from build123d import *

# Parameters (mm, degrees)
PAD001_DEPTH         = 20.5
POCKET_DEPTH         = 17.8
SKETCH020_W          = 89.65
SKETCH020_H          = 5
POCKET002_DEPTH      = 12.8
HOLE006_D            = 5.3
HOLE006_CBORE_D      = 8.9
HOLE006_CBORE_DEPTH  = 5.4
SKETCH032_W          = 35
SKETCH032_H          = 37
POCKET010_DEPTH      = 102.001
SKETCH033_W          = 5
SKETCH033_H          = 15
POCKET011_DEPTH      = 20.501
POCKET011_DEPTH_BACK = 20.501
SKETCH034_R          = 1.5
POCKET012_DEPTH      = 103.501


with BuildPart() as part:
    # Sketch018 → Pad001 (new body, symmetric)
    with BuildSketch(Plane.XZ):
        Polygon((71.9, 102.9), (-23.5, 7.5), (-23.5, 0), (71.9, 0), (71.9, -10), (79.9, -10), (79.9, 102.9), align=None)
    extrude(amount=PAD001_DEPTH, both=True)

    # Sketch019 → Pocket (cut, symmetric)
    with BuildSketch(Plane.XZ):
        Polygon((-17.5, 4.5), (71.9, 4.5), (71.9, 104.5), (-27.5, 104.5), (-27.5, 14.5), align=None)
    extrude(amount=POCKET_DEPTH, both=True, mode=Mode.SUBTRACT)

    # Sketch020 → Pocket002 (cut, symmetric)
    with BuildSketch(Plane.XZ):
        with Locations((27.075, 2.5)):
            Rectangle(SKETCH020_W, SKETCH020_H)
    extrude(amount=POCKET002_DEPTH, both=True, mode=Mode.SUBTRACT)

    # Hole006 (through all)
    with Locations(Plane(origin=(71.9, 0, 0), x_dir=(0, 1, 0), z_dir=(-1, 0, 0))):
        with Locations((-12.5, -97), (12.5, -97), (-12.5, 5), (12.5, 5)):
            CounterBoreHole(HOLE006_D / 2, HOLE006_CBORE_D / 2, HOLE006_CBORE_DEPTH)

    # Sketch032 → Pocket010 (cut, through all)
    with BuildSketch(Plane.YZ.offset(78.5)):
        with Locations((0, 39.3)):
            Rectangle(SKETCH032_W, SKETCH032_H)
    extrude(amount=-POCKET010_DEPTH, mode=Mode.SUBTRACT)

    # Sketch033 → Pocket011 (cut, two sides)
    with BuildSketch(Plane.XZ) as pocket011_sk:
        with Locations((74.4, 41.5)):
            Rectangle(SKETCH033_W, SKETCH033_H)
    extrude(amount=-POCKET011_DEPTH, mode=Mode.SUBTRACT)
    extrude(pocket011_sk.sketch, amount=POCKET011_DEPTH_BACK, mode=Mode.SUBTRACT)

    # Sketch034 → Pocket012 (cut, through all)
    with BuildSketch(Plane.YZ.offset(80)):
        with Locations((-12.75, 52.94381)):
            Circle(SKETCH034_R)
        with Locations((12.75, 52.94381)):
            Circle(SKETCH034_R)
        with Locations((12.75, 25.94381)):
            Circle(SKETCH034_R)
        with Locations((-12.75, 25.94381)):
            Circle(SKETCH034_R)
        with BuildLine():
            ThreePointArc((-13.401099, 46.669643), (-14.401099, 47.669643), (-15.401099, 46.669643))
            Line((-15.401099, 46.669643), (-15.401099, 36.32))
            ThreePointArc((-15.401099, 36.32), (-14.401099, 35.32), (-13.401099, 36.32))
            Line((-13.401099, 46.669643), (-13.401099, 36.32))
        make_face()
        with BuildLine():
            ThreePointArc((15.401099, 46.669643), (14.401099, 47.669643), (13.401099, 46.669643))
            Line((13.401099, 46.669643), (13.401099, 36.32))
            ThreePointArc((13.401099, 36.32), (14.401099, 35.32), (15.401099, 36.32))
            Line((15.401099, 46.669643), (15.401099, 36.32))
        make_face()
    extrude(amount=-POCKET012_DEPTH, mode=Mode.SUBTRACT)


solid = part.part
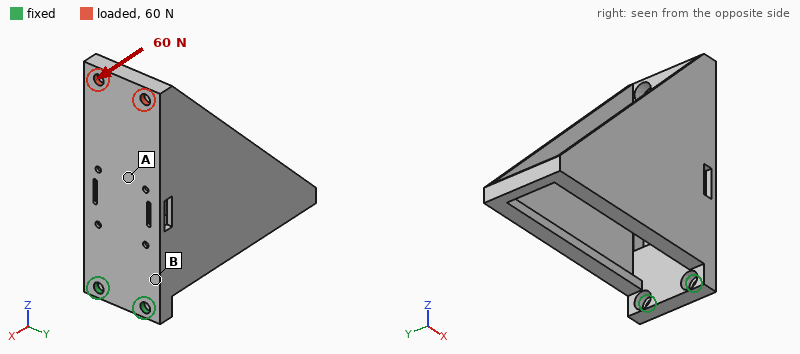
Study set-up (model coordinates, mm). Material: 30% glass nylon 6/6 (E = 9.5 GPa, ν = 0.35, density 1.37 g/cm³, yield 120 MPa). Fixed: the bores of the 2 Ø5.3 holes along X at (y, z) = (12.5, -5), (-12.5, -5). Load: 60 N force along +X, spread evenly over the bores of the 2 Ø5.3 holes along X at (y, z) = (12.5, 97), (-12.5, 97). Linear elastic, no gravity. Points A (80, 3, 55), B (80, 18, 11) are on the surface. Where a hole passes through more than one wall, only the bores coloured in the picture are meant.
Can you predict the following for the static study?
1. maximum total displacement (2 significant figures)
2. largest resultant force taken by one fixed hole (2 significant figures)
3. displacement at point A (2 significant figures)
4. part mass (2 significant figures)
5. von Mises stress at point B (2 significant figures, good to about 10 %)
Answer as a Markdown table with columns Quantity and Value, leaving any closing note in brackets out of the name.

| Quantity | Value |
|---|---|
| maximum total displacement | 1.5 mm |
| largest resultant force taken by one fixed hole | 51 N |
| displacement at point A | 0.82 mm |
| part mass | 83 g |
| von Mises stress at point B | 5.4 MPa |
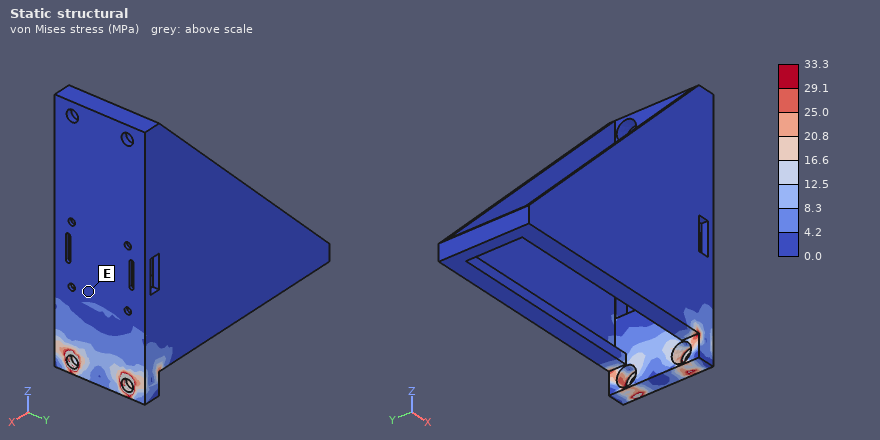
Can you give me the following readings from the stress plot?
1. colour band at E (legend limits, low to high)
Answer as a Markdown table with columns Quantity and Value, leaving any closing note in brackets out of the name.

| Quantity | Value |
|---|---|
| colour band at E | 0.0 to 4.2 MPa |
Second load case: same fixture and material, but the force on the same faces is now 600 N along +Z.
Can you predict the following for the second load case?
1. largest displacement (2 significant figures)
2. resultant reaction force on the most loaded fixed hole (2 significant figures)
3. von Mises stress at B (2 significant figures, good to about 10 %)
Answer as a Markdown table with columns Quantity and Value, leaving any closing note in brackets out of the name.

| Quantity | Value |
|---|---|
| largest displacement | 0.18 mm |
| resultant reaction force on the most loaded fixed hole | 300 N |
| von Mises stress at B | 4.5 MPa |
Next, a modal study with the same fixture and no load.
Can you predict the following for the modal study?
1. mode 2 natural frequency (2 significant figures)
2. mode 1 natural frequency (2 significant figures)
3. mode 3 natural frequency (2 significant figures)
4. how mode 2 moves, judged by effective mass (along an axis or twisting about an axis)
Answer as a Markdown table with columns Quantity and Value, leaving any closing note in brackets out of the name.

| Quantity | Value |
|---|---|
| mode 2 natural frequency | 330 Hz |
| mode 1 natural frequency | 180 Hz |
| mode 3 natural frequency | 670 Hz |
| how mode 2 moves, judged by effective mass | along Y |
